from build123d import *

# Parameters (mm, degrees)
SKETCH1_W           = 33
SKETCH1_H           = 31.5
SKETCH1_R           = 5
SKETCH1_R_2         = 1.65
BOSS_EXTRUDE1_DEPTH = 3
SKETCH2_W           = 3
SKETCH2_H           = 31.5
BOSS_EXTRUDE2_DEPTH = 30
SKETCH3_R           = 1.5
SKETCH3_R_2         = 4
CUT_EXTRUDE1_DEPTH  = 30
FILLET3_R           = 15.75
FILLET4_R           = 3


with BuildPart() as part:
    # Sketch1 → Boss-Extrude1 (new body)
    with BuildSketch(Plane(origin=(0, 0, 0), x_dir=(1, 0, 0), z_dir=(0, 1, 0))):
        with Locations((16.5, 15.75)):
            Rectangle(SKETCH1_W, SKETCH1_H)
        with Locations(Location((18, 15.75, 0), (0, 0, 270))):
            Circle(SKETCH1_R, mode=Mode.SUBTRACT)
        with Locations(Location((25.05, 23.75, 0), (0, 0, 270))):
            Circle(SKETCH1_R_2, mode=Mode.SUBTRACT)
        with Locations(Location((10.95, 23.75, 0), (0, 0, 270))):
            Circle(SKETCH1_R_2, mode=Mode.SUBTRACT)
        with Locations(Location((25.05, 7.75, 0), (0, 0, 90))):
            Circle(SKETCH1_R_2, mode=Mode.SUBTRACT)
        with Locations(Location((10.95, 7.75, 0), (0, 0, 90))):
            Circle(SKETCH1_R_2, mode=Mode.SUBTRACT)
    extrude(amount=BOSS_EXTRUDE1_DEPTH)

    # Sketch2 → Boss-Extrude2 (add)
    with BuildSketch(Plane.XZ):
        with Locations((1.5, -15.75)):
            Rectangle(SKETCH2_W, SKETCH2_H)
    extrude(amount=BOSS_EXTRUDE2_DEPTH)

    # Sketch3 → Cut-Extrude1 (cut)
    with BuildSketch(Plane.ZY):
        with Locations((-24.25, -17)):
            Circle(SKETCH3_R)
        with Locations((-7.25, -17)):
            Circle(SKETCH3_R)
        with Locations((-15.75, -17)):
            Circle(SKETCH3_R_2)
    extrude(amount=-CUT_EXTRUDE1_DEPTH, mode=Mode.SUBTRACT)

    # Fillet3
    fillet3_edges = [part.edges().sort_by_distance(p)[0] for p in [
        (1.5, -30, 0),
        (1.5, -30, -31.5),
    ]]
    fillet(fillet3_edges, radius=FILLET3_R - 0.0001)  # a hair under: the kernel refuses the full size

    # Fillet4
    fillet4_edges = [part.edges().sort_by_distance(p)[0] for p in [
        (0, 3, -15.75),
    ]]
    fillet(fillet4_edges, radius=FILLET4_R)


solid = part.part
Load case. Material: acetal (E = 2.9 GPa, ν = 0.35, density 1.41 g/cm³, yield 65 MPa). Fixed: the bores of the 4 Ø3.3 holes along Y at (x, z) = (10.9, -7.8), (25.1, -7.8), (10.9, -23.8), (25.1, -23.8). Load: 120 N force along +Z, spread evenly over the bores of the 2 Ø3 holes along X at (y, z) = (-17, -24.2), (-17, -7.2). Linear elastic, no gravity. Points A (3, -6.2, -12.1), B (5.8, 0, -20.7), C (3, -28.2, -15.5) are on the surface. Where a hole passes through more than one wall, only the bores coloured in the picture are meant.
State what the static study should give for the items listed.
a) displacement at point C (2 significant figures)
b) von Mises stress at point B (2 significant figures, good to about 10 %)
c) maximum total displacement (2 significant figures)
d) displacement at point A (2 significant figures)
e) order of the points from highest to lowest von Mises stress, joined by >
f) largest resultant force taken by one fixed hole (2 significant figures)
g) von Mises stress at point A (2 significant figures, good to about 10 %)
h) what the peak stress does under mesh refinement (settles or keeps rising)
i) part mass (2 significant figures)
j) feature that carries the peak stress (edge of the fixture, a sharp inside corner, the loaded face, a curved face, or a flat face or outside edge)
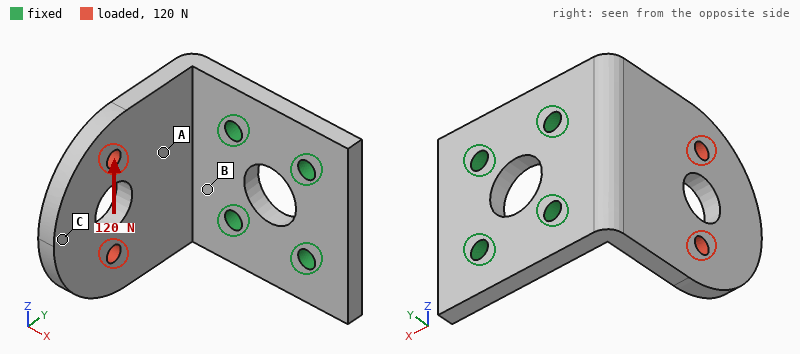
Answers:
0.64 mm
16 MPa
0.67 mm
0.19 mm
B > A > C
140 N
8.3 MPa
keeps rising
7.1 g
edge of the fixture
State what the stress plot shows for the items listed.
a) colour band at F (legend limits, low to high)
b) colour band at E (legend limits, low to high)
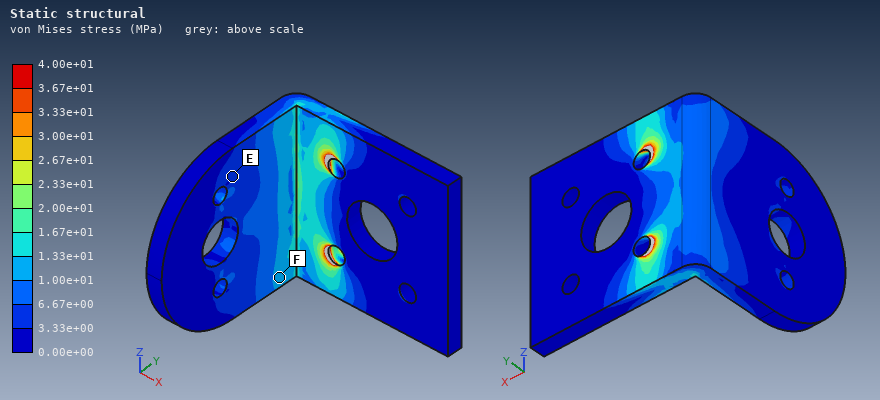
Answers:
1.00e+01 to 1.33e+01 MPa
3.33e+00 to 6.67e+00 MPa
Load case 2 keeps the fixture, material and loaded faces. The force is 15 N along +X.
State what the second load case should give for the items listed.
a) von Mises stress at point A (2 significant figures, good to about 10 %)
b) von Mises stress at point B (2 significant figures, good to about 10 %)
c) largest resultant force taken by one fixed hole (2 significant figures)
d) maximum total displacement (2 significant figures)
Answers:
3.1 MPa
5.4 MPa
7.8 N
0.65 mm
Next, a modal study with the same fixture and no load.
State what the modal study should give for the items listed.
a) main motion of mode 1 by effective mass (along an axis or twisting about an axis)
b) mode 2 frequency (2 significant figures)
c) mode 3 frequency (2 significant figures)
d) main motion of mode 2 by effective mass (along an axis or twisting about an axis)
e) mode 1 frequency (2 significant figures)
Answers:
along X
1400 Hz
2100 Hz
along Z
600 Hz
